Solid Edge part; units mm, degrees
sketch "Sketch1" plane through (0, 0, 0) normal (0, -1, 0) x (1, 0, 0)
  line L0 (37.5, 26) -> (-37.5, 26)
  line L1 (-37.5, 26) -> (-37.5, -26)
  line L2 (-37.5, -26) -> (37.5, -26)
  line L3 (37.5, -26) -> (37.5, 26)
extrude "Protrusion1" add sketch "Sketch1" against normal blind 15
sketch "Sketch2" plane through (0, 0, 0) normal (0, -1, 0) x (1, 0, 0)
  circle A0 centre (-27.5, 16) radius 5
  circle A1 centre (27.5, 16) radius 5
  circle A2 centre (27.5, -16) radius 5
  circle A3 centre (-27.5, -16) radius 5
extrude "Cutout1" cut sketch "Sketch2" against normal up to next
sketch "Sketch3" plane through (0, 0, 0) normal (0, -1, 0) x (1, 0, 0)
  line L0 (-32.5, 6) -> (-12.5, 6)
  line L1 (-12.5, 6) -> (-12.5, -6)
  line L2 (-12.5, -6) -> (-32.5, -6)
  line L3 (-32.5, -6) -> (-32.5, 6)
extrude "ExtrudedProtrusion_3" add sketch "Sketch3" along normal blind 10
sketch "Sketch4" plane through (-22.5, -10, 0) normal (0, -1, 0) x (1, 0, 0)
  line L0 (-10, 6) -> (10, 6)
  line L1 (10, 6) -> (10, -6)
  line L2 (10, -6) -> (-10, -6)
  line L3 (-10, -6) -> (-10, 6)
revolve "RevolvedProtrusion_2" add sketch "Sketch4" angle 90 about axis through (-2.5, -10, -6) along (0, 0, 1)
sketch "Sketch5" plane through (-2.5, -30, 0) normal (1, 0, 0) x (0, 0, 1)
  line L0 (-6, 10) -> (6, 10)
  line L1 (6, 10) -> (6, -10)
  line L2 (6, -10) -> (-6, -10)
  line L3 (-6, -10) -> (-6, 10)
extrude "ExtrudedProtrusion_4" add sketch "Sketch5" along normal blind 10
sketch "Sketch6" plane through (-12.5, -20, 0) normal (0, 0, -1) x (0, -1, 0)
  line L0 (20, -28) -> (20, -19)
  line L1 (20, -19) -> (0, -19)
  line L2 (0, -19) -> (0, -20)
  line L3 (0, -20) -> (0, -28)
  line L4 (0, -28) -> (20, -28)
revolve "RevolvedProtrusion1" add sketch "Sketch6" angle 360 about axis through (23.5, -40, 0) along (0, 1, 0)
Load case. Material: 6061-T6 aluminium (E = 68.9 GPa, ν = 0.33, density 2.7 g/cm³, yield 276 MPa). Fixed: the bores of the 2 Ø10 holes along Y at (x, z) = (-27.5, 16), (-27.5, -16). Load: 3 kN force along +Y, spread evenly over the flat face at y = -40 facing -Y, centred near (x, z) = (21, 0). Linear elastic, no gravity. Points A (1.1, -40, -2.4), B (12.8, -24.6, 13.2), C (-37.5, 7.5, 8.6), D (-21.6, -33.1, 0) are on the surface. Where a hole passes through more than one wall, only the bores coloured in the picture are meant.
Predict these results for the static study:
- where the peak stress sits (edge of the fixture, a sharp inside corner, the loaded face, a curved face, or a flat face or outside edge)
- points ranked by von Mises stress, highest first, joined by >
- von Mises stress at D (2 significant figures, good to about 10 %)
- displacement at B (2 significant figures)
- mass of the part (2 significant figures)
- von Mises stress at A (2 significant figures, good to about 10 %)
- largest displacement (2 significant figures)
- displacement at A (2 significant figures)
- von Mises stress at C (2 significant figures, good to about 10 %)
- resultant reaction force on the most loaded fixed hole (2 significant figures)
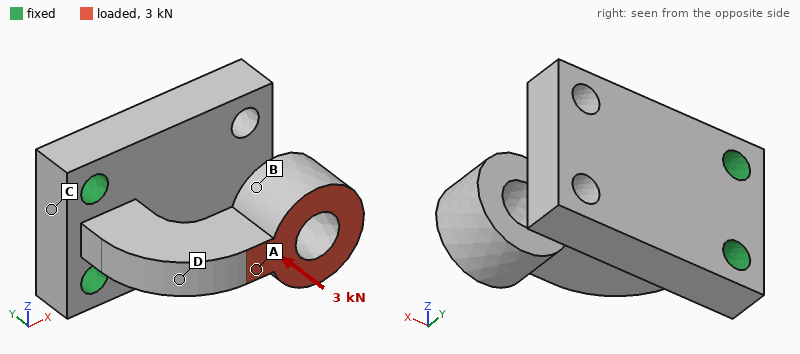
a curved face
D > A > C > B
92 MPa
0.37 mm
220 g
73 MPa
0.75 mm
0.36 mm
43 MPa
1.5 kN
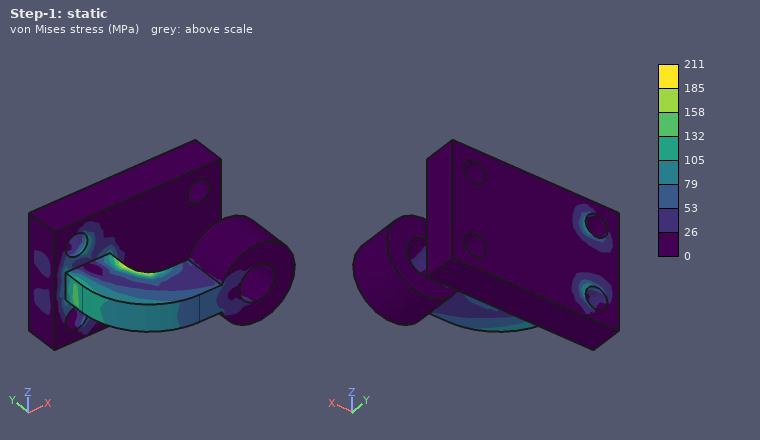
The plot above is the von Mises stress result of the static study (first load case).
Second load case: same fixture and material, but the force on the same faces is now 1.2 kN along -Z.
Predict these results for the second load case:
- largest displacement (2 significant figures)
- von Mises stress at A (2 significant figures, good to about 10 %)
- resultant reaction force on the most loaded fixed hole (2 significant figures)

0.80 mm
38 MPa
2.7 kN
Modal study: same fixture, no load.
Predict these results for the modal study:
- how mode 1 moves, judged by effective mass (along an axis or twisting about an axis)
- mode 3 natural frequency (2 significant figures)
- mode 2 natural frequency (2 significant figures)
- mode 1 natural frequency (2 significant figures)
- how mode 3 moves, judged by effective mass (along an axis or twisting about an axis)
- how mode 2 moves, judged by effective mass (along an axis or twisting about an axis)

along Z
3300 Hz
1700 Hz
1100 Hz
along Y
along Y
